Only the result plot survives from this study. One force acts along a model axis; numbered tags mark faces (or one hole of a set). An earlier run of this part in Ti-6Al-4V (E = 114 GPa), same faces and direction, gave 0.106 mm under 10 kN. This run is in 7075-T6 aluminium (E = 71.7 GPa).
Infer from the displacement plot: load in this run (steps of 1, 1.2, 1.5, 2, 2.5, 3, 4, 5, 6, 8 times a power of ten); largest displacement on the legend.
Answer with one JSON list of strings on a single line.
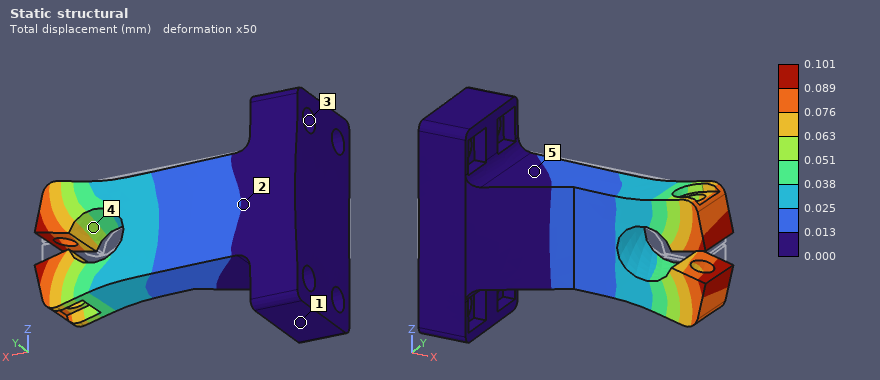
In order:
["6 kN", "0.101 mm"]
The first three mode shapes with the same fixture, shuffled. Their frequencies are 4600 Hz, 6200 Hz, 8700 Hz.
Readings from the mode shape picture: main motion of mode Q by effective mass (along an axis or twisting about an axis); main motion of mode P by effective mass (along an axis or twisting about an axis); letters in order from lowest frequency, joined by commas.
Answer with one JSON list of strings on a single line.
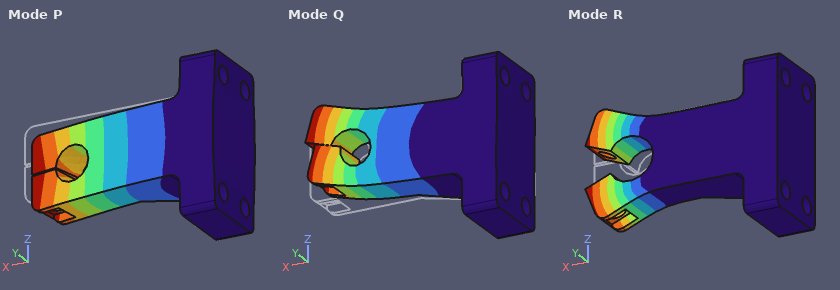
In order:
["along Z", "along Y", "P, Q, R"]
